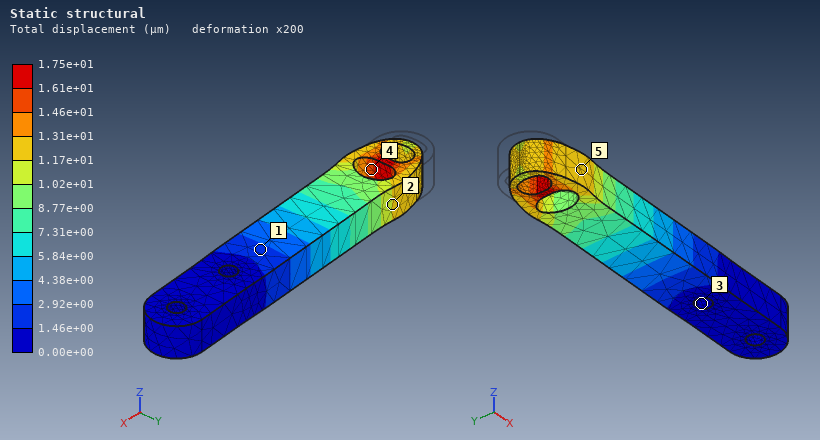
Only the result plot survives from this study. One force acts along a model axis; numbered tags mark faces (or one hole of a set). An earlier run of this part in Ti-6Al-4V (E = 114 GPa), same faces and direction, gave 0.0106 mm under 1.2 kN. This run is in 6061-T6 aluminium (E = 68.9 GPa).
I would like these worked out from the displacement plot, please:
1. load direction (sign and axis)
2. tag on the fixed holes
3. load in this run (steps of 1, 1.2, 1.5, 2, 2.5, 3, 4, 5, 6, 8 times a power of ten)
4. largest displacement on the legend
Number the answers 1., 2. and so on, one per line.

1. +X
2. 3
3. 1.2 kN
4. 1.75e+01 µm
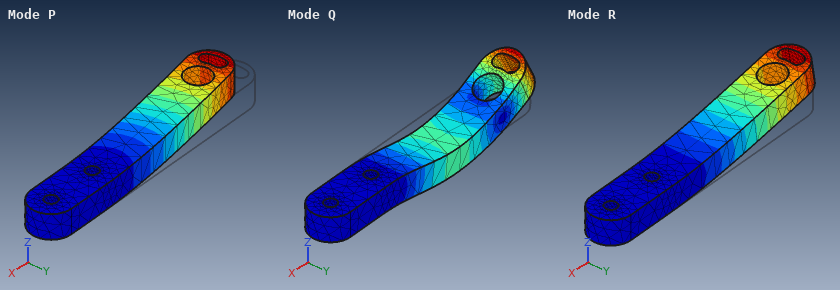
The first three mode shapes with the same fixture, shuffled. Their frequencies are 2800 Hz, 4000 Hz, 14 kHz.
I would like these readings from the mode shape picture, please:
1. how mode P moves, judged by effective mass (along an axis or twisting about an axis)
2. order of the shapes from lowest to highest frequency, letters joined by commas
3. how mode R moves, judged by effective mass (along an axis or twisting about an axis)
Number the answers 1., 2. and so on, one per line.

1. along Y
2. R, P, Q
3. along Z
